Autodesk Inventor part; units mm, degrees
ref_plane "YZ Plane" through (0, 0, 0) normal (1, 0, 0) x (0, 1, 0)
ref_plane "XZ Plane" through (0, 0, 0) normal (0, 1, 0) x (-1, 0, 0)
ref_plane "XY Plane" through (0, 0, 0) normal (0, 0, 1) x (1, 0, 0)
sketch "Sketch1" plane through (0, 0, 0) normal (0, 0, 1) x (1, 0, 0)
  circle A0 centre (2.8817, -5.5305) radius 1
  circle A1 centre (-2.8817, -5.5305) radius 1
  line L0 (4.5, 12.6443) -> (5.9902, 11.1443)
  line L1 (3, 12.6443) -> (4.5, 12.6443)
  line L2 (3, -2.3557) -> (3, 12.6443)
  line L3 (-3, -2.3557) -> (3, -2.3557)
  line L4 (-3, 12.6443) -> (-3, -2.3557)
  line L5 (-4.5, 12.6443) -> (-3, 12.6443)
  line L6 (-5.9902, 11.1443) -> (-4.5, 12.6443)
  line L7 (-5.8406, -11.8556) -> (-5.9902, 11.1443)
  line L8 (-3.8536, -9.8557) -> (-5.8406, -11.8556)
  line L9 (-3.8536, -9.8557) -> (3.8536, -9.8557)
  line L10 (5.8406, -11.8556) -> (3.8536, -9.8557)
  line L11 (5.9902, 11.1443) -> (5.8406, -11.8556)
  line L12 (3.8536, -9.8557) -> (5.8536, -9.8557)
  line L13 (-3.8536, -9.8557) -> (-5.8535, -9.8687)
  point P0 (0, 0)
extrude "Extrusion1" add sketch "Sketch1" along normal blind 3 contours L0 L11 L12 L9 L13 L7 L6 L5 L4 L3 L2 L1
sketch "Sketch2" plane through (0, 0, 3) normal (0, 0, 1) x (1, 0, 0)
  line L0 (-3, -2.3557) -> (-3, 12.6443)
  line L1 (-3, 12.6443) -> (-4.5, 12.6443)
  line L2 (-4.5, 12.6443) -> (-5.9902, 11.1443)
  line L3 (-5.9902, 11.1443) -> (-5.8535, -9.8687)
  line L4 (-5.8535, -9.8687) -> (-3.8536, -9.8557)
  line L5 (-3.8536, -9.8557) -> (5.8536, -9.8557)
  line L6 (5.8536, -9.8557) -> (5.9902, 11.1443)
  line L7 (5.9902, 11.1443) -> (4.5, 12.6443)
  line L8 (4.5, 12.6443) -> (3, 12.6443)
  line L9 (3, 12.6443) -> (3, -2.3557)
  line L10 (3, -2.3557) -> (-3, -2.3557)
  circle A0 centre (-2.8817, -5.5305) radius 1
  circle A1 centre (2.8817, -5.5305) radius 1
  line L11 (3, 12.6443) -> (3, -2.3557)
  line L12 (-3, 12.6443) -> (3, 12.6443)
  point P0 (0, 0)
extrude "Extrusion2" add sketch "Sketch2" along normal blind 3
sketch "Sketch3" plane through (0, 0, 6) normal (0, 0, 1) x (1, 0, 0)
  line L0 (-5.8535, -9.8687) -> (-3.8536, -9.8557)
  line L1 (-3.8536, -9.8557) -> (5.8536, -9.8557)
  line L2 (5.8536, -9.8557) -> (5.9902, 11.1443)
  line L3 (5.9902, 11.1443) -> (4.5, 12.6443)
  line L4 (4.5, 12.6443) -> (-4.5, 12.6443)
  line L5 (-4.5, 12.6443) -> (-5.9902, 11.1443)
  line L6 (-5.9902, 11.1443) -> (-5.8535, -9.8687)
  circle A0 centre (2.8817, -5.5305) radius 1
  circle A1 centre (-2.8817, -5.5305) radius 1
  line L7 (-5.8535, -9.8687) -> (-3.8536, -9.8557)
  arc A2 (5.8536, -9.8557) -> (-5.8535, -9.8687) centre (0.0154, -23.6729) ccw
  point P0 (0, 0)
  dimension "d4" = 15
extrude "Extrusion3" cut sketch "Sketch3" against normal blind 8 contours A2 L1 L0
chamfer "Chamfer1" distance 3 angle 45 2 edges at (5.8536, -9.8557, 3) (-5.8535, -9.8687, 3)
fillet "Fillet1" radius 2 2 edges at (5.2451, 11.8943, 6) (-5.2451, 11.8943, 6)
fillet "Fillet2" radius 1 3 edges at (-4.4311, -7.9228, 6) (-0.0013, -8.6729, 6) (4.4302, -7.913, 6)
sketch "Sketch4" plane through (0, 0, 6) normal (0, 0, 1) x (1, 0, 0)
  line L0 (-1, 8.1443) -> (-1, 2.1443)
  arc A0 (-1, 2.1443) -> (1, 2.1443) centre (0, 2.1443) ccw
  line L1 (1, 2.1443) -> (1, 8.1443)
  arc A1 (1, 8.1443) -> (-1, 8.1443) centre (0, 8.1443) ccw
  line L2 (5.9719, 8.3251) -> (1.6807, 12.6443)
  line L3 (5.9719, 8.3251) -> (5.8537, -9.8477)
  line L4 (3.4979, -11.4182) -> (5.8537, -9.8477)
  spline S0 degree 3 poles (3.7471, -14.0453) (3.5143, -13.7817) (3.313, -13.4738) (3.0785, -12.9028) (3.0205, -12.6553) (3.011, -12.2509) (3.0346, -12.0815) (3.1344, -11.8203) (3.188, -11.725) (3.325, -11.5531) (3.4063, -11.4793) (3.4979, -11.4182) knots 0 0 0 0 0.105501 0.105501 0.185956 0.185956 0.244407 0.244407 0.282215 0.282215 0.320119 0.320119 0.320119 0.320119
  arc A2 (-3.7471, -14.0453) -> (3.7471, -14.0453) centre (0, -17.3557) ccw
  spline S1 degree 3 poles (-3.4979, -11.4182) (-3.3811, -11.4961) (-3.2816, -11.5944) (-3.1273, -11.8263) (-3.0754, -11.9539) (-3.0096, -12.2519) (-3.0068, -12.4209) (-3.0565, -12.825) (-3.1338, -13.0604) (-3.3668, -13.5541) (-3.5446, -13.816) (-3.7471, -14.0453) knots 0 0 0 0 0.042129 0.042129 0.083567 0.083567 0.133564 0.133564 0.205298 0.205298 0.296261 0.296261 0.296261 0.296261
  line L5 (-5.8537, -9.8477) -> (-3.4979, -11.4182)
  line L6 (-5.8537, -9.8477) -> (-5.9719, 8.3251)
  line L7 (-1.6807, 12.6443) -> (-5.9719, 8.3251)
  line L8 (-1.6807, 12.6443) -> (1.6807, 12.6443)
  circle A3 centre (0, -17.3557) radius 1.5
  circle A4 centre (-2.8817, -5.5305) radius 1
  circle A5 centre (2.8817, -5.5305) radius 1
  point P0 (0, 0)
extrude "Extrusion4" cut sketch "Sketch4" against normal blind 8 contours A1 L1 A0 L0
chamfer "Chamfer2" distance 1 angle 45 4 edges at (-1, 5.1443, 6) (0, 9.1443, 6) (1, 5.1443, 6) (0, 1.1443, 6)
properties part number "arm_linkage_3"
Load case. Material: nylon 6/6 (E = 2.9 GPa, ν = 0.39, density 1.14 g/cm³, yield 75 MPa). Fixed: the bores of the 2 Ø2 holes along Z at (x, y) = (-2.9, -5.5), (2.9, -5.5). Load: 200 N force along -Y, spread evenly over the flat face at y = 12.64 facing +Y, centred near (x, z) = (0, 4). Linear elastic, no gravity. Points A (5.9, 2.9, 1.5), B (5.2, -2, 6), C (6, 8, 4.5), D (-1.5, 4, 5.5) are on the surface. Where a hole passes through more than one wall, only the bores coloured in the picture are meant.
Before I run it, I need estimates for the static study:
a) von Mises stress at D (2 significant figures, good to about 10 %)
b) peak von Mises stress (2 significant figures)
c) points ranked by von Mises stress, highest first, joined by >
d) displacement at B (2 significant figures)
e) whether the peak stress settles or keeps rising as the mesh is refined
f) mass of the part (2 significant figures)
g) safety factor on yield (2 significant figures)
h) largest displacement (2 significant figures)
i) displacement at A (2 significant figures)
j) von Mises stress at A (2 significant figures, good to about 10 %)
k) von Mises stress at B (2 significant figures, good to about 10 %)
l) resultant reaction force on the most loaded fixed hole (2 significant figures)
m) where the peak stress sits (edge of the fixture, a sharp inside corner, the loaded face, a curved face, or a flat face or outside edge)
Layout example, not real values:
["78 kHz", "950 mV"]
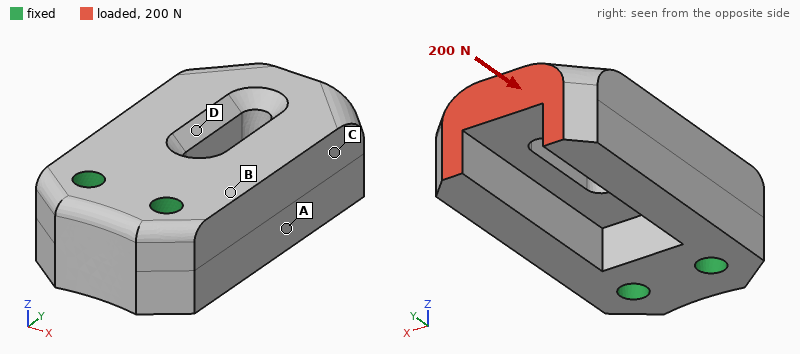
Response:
["7.4 MPa", "16 MPa", "D > B > A > C", "8.8 µm", "settles", "1.3 g", "4.6", "47 µm", "16 µm", "2.4 MPa", "4.6 MPa", "100 N", "a curved face"]
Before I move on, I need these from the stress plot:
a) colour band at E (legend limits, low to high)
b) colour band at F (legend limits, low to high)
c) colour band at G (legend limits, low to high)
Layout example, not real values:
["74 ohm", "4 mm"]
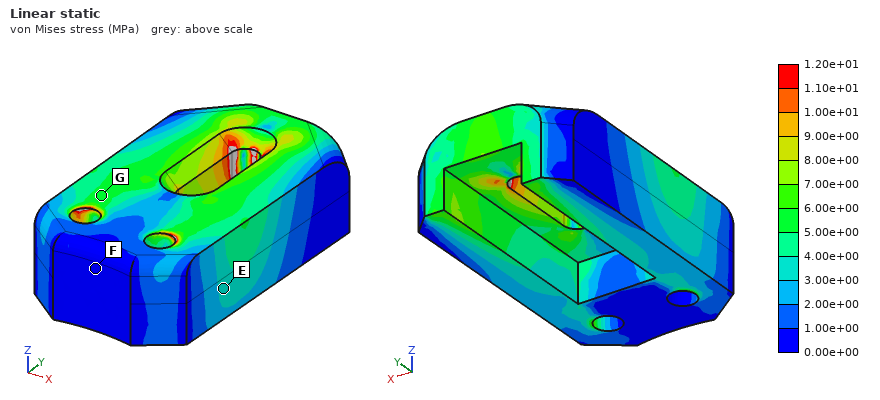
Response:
["3.00e+00 to 4.00e+00 MPa", "0.00e+00 to 1.00e+00 MPa", "5.00e+00 to 6.00e+00 MPa"]
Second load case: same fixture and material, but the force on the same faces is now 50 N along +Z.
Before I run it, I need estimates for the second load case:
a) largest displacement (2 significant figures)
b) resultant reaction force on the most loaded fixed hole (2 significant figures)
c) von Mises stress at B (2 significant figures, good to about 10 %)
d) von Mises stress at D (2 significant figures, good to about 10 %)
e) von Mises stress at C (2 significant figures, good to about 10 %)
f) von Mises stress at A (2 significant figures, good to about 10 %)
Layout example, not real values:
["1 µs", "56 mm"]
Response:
["0.28 mm", "28 N", "13 MPa", "7.7 MPa", "2.6 MPa", "7.4 MPa"]
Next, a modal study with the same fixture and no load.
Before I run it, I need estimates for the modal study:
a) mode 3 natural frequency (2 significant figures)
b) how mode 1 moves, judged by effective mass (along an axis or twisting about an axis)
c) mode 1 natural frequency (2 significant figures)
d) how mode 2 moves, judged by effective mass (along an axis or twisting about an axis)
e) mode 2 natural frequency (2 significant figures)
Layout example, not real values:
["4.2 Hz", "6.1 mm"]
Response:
["8200 Hz", "along Z", "4500 Hz", "along X", "5600 Hz"]
